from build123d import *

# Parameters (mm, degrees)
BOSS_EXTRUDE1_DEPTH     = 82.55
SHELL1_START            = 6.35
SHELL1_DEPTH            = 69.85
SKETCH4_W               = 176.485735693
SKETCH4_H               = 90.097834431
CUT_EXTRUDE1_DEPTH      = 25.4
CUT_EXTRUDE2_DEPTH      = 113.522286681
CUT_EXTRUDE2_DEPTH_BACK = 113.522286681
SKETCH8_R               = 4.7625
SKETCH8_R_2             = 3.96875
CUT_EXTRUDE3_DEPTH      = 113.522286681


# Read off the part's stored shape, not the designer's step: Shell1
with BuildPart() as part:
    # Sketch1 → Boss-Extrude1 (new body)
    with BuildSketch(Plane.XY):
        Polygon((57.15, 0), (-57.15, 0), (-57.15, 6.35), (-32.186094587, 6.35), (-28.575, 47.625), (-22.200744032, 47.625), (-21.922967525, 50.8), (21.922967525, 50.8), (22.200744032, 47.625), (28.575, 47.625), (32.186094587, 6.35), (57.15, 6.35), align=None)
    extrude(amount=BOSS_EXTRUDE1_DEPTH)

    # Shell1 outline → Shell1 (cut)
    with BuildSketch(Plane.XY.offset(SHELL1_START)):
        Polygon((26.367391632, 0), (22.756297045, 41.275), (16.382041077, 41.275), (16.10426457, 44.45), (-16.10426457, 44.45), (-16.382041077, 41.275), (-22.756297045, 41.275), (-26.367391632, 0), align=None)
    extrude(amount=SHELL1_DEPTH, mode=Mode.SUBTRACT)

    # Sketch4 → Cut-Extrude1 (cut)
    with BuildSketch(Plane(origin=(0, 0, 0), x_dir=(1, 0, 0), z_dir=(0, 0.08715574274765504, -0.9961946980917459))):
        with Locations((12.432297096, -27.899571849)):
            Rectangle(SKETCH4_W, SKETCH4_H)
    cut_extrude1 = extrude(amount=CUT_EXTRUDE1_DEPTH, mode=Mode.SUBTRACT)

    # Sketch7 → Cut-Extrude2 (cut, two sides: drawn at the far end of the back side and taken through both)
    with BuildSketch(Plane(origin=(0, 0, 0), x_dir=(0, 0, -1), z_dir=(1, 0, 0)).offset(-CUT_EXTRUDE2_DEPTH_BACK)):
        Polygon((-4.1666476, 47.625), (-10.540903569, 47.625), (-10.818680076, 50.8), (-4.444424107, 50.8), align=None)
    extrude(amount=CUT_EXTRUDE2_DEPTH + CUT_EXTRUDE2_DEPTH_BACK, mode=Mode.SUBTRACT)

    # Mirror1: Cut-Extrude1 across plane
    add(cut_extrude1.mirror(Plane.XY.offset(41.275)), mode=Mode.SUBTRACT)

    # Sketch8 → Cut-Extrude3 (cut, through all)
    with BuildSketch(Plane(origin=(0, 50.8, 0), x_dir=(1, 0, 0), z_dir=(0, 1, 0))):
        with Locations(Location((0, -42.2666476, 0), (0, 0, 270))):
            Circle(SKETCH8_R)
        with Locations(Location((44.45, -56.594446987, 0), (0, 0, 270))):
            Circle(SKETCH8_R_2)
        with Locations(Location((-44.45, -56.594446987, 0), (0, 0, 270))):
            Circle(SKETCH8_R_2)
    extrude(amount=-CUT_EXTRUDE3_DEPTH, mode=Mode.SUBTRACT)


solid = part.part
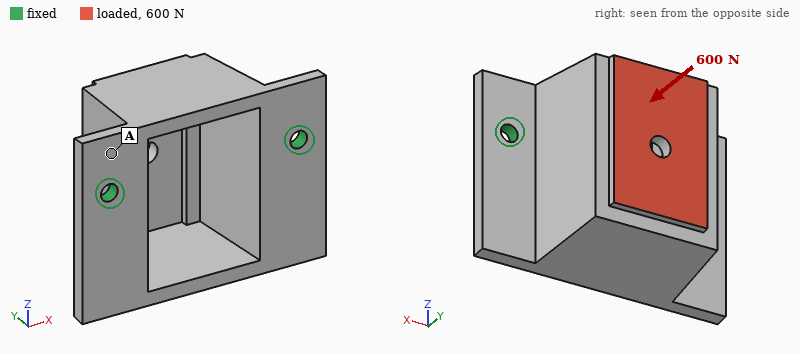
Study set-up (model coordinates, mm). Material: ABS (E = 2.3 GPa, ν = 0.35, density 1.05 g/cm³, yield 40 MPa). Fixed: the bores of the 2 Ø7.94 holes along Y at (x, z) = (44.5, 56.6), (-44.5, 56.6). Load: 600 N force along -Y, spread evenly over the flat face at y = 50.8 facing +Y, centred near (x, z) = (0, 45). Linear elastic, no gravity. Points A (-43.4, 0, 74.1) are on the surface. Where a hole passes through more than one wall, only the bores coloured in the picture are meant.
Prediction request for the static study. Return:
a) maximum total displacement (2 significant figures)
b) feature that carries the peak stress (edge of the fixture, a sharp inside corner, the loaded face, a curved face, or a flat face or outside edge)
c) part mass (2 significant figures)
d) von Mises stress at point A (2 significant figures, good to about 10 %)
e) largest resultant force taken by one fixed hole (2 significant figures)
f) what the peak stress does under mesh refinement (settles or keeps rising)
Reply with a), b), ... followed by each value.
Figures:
a) 0.87 mm
b) edge of the fixture
c) 120 g
d) 1.9 MPa
e) 320 N
f) keeps rising
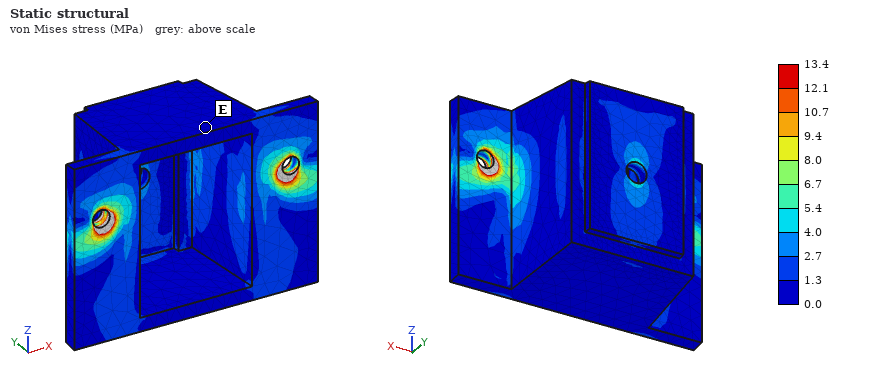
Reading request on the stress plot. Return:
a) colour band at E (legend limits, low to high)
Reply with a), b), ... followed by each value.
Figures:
a) 0.0 to 1.3 MPa
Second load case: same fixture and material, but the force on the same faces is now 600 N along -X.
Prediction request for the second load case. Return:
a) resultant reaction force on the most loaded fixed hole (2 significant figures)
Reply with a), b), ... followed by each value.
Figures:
a) 490 N
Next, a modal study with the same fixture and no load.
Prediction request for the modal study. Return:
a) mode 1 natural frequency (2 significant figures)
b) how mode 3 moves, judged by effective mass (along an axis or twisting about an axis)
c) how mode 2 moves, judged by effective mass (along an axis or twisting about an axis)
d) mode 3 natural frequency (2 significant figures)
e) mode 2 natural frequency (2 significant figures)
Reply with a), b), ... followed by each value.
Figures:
a) 290 Hz
b) along X
c) along X
d) 1000 Hz
e) 860 Hz
